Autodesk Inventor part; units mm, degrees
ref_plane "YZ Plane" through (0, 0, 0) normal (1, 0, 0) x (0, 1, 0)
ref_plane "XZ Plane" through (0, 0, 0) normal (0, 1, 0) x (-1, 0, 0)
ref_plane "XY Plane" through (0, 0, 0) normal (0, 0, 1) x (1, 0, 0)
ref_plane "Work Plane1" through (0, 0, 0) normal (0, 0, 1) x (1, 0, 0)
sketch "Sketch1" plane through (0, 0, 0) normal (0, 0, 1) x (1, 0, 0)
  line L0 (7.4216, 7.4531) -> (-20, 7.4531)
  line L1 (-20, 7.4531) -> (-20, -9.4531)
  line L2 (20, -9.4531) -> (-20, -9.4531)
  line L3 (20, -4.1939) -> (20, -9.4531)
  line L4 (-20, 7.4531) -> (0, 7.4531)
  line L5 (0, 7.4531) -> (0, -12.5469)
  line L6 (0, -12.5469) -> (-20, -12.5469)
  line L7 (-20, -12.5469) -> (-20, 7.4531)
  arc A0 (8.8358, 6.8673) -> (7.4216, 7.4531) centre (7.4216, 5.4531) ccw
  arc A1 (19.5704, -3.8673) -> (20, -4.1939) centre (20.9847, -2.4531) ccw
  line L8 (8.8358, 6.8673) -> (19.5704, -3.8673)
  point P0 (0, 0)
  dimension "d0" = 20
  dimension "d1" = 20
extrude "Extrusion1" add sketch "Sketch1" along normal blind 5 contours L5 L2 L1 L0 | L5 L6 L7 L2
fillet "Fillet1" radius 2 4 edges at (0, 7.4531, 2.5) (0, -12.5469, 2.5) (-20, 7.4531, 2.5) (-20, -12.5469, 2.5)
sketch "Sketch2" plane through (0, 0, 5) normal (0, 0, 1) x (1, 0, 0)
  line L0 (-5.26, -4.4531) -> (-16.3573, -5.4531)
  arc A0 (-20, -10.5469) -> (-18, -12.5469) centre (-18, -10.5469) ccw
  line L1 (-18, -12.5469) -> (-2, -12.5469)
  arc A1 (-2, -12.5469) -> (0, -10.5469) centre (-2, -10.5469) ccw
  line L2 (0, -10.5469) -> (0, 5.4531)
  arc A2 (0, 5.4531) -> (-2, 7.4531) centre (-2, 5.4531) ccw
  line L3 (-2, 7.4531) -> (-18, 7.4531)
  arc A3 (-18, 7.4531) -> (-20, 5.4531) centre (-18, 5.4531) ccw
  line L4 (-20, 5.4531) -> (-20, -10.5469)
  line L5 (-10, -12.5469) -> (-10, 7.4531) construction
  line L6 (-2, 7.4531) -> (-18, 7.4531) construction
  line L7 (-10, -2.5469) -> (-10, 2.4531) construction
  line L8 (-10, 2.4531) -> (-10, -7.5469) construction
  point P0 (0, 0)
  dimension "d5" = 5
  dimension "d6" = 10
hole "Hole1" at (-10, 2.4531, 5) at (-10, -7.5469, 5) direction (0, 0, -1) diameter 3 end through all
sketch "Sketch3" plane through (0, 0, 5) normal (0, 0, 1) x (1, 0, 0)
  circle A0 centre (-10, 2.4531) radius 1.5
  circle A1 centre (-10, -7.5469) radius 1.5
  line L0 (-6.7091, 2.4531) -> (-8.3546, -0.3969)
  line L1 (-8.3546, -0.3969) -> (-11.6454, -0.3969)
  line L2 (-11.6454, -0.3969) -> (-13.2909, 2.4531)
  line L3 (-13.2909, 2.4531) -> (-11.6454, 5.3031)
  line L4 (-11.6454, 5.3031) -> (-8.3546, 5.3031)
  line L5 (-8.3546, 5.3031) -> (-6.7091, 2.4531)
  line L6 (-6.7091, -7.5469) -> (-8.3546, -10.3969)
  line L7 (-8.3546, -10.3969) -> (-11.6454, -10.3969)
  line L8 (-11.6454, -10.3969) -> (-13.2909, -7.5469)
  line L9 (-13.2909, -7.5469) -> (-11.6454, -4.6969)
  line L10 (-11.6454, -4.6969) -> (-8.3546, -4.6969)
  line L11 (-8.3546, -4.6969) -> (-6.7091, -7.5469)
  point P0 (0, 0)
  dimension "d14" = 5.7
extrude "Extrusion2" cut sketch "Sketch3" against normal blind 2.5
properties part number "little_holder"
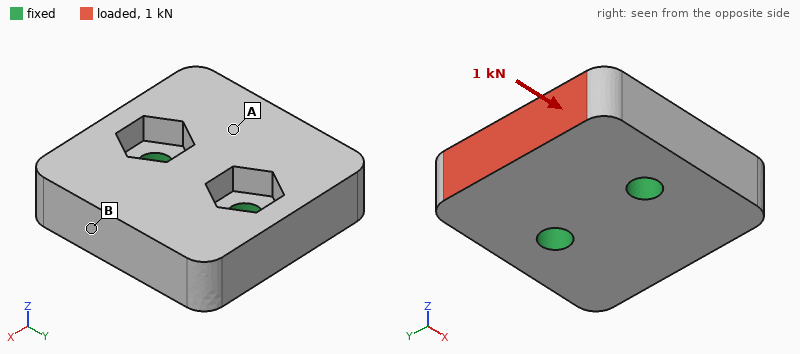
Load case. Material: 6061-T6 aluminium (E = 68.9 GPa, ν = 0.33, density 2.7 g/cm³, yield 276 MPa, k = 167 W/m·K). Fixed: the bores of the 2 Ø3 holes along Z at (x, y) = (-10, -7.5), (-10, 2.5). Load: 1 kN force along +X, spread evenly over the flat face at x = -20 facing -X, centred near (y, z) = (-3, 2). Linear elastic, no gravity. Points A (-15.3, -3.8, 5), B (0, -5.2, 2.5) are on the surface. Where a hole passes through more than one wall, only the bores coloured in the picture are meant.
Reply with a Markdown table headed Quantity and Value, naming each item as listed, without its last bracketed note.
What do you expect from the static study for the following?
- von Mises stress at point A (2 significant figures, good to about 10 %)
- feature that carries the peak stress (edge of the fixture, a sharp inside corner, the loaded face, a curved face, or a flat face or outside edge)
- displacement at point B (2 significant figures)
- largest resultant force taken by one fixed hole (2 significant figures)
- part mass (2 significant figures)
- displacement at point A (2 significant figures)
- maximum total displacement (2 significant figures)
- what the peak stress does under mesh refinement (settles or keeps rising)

| Quantity | Value |
|---|---|
| von Mises stress at point A | 16 MPa |
| feature that carries the peak stress | edge of the fixture |
| displacement at point B | 5.4 µm |
| largest resultant force taken by one fixed hole | 510 N |
| part mass | 4.9 g |
| displacement at point A | 5.7 µm |
| maximum total displacement | 9.2 µm |
| what the peak stress does under mesh refinement | keeps rising |
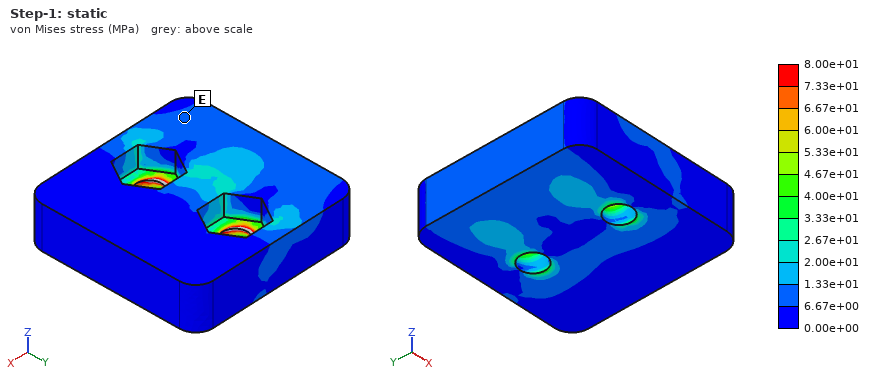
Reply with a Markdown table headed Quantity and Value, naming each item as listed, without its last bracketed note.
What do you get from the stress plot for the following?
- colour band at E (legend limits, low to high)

| Quantity | Value |
|---|---|
| colour band at E | 6.67e+00 to 1.33e+01 MPa |
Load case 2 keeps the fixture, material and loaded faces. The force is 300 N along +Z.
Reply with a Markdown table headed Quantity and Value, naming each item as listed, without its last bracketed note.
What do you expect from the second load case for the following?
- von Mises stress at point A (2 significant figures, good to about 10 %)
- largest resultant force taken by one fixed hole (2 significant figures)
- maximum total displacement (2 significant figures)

| Quantity | Value |
|---|---|
| von Mises stress at point A | 23 MPa |
| largest resultant force taken by one fixed hole | 150 N |
| maximum total displacement | 22 µm |
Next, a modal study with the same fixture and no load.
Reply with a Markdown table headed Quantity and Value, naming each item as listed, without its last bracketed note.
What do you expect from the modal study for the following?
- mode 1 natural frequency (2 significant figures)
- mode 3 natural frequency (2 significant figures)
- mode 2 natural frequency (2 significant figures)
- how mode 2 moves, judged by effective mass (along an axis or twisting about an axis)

| Quantity | Value |
|---|---|
| mode 1 natural frequency | 17 kHz |
| mode 3 natural frequency | 34 kHz |
| mode 2 natural frequency | 31 kHz |
| how mode 2 moves, judged by effective mass | along Z |
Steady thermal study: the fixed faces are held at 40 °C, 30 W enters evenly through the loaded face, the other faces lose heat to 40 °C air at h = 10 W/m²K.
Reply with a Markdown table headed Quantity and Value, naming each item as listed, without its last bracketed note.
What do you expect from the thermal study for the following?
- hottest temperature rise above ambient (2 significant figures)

| Quantity | Value |
|---|---|
| hottest temperature rise above ambient | 24 K |
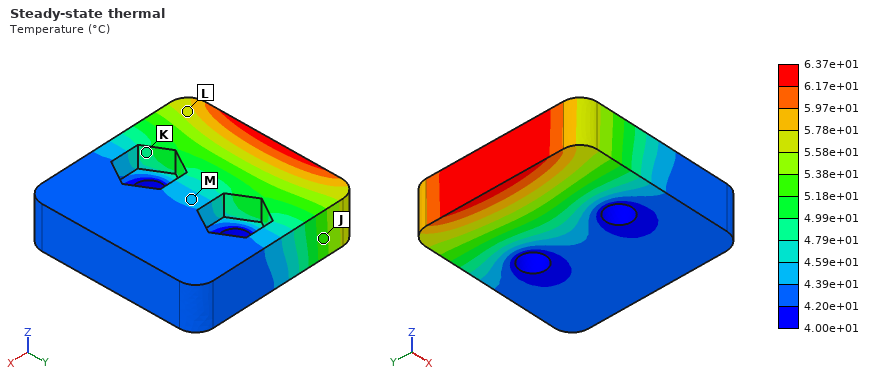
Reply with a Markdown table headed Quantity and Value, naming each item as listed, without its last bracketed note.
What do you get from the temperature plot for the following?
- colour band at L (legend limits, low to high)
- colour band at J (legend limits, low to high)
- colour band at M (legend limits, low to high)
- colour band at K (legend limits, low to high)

| Quantity | Value |
|---|---|
| colour band at L | 5.58e+01 to 5.78e+01 °C |
| colour band at J | 5.18e+01 to 5.38e+01 °C |
| colour band at M | 4.39e+01 to 4.59e+01 °C |
| colour band at K | 4.79e+01 to 4.99e+01 °C |
